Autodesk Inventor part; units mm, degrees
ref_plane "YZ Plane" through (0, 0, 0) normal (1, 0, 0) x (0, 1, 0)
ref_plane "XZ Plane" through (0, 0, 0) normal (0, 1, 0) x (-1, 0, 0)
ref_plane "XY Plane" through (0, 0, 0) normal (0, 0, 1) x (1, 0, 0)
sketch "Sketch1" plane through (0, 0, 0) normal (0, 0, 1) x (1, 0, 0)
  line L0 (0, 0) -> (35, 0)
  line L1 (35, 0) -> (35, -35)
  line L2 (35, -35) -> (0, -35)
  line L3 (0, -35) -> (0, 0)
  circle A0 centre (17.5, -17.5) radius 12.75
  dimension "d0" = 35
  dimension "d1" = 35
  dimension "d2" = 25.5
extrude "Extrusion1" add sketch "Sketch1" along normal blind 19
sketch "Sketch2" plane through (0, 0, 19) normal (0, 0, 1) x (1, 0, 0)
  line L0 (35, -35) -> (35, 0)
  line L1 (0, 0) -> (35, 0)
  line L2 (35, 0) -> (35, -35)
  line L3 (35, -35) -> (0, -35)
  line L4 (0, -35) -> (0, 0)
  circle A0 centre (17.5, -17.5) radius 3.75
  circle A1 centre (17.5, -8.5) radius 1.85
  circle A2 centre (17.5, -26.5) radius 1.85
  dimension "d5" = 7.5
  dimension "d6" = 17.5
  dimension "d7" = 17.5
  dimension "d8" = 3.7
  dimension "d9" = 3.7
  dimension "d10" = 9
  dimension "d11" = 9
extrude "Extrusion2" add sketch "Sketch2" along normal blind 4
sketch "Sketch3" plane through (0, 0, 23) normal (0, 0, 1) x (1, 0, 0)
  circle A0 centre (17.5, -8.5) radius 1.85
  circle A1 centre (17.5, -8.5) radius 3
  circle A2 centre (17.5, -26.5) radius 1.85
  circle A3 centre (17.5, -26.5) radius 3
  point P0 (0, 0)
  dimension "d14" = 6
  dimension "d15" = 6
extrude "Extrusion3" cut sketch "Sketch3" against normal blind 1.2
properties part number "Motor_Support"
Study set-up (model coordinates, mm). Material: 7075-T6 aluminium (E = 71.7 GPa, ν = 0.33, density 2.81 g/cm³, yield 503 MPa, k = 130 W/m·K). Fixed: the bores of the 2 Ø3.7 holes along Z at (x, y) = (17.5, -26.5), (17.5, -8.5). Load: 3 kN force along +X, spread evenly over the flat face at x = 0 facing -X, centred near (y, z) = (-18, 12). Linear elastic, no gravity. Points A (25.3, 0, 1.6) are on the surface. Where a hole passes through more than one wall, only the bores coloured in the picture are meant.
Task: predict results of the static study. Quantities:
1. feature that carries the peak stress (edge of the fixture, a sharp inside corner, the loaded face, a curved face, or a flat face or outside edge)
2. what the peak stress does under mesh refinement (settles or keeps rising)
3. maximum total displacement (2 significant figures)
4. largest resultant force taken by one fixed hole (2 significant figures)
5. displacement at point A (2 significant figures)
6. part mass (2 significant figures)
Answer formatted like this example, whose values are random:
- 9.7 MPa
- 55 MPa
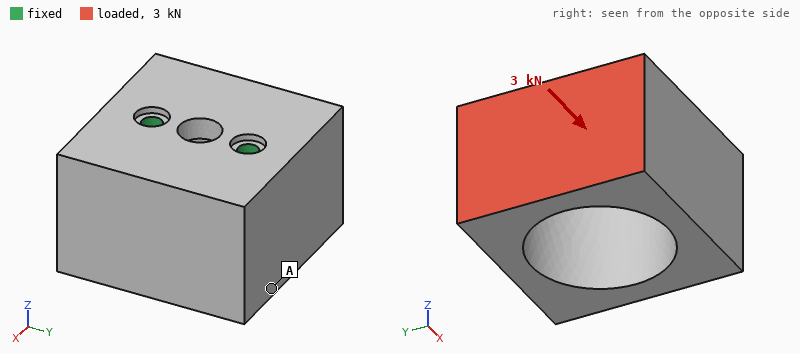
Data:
- edge of the fixture
- keeps rising
- 0.22 mm
- 1.5 kN
- 0.16 mm
- 51 g
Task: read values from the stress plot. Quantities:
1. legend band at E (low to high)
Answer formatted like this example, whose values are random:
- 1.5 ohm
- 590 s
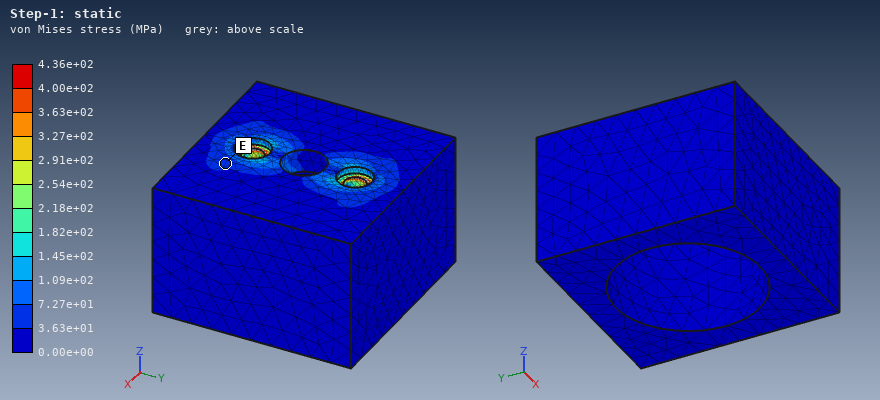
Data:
- 3.63e+01 to 7.27e+01 MPa
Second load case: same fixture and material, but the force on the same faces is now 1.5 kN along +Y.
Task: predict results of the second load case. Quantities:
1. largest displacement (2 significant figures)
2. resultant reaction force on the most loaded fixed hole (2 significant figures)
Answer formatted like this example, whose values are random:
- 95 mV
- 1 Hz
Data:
- 29 µm
- 1.6 kN
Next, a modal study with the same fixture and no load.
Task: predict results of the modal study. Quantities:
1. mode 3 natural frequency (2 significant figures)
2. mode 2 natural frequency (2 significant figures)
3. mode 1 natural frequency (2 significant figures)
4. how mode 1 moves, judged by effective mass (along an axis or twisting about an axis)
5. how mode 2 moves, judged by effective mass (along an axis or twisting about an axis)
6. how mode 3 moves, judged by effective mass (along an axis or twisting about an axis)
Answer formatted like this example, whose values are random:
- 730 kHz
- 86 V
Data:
- 11 kHz
- 7000 Hz
- 2600 Hz
- along X
- along Y
- twisting about Z
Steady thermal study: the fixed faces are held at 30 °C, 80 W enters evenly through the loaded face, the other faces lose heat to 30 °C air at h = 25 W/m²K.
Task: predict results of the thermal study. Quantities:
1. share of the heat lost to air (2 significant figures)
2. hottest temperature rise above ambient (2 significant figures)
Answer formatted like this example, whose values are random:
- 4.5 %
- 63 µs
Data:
- 5.3 %
- 52 K
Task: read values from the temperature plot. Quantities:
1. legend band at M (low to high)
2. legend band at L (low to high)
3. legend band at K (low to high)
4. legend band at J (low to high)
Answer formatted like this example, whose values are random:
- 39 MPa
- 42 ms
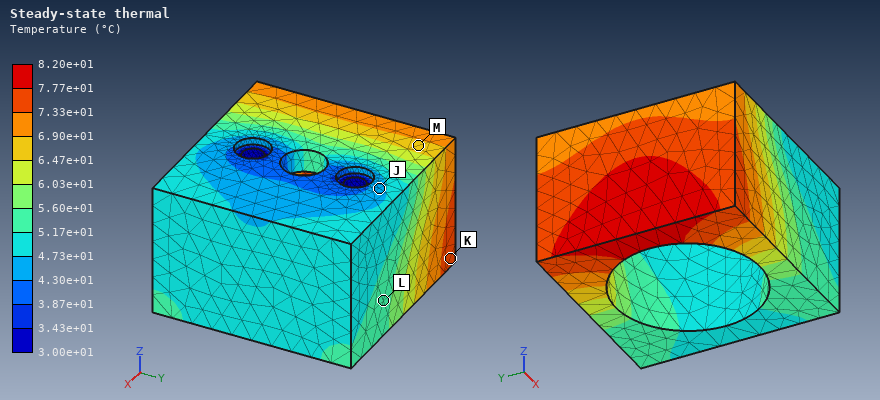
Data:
- 6.47e+01 to 6.90e+01 °C
- 5.17e+01 to 5.60e+01 °C
- 7.33e+01 to 7.77e+01 °C
- 4.30e+01 to 4.73e+01 °C
